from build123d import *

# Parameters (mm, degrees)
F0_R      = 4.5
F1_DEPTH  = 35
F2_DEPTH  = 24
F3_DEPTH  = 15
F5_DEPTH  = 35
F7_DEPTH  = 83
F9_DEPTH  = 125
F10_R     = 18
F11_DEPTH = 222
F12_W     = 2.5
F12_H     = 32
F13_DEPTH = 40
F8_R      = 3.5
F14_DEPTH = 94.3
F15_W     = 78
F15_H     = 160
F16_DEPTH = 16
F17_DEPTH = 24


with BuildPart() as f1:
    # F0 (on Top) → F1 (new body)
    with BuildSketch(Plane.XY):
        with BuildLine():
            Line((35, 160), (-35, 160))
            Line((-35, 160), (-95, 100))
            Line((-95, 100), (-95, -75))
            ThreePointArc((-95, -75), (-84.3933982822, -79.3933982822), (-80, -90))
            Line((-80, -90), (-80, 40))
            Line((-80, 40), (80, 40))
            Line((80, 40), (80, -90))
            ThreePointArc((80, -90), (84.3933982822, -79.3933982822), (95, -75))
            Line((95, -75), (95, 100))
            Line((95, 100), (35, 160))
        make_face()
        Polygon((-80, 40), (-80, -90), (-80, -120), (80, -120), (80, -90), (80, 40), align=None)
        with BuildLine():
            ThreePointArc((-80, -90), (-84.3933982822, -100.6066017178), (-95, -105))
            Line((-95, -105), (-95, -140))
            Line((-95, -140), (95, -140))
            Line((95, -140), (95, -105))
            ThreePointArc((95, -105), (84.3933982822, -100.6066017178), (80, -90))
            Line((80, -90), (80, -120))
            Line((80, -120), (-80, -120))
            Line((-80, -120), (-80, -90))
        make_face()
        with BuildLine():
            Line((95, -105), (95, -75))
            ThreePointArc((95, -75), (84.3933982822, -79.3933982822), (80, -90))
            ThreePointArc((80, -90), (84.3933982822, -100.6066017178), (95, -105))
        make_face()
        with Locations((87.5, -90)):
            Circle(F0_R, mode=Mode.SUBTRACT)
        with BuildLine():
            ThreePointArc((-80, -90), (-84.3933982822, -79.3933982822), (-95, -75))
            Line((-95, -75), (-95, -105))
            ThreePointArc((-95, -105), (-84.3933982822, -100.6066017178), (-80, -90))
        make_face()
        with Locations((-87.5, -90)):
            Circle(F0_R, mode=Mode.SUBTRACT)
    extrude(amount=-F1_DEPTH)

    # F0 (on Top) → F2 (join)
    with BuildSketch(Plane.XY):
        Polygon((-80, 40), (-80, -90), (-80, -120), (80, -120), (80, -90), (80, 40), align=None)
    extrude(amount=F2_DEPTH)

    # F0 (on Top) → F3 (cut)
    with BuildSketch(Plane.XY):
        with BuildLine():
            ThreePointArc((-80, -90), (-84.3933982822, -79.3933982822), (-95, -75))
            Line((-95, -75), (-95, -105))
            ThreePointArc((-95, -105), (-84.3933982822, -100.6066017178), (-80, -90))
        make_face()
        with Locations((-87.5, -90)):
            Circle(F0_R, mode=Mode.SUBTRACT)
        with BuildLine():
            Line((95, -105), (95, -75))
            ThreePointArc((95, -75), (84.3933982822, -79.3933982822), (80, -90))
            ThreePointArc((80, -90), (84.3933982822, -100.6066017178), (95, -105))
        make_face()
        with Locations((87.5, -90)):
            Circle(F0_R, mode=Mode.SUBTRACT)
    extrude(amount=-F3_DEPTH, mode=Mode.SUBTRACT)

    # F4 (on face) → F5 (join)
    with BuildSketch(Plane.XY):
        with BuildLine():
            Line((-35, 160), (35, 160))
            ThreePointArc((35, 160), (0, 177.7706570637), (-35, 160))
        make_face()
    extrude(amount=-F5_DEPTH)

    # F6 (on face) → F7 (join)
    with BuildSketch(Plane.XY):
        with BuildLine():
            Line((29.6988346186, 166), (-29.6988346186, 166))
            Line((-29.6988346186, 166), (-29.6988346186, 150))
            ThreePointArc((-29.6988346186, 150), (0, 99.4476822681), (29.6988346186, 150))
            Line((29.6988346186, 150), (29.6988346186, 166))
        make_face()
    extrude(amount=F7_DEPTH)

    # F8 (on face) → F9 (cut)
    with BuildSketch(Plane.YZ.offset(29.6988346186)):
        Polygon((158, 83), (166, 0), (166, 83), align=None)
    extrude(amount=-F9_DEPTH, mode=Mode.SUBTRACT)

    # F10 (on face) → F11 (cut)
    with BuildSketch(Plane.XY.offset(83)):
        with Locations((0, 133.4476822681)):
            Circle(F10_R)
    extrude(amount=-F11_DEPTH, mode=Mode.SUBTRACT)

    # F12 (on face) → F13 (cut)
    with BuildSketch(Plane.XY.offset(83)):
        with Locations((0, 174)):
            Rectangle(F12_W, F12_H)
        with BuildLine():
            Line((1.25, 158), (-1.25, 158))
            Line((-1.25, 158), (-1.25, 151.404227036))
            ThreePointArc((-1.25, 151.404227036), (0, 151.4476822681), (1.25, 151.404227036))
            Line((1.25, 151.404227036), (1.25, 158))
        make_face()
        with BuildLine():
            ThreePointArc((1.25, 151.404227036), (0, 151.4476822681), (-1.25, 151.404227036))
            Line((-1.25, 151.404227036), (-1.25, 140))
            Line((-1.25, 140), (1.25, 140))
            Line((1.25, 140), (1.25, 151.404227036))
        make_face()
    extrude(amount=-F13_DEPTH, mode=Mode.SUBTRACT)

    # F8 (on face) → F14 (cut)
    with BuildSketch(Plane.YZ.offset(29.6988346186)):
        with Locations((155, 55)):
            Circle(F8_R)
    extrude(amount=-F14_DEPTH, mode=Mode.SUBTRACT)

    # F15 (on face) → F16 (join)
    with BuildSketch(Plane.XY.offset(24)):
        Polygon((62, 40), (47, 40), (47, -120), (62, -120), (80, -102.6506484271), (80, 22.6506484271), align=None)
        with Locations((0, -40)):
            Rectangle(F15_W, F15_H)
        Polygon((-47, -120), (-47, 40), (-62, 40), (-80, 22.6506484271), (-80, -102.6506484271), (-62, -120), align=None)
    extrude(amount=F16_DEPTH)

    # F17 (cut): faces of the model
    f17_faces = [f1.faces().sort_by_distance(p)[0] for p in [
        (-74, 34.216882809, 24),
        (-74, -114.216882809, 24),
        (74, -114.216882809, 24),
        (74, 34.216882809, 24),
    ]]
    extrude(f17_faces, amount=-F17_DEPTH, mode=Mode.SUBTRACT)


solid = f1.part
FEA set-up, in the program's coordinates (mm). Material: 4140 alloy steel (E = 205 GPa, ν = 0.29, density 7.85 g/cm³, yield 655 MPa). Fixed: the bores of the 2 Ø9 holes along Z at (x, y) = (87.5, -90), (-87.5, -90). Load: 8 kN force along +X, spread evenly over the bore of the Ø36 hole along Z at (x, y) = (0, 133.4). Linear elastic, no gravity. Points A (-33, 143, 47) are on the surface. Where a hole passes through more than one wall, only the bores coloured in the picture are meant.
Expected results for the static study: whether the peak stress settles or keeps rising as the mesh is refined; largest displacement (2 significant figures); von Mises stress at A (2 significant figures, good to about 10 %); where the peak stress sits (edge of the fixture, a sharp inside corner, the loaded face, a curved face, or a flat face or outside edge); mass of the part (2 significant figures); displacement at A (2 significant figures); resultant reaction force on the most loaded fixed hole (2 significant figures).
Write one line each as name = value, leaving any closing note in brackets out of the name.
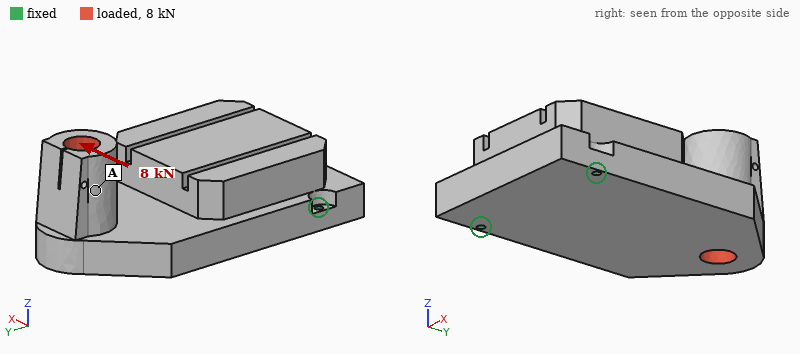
whether the peak stress settles or keeps rising as the mesh is refined = keeps rising
largest displacement = 38 µm
von Mises stress at A = 3.1 MPa
where the peak stress sits = edge of the fixture
mass of the part = 24 kg
displacement at A = 28 µm
resultant reaction force on the most loaded fixed hole = 11 kN
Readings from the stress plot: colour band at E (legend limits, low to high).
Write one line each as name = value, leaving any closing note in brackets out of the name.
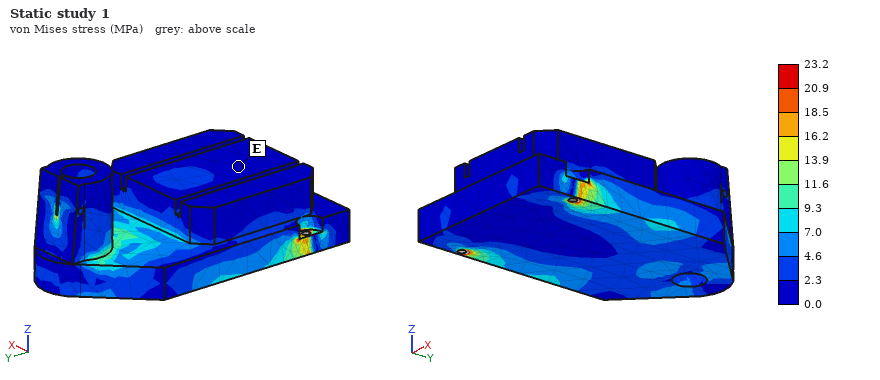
colour band at E = 0.0 to 2.3 MPa
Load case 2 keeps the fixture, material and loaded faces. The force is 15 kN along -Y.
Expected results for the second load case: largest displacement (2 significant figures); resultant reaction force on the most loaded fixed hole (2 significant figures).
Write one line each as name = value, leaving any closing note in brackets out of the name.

largest displacement = 0.27 mm
resultant reaction force on the most loaded fixed hole = 7.5 kN
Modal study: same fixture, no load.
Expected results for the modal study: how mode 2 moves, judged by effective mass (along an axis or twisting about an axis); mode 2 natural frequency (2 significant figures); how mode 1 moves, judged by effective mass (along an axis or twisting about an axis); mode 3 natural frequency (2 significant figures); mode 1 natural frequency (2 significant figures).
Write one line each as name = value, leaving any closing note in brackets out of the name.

how mode 2 moves, judged by effective mass = along X
mode 2 natural frequency = 1400 Hz
how mode 1 moves, judged by effective mass = along Z
mode 3 natural frequency = 1600 Hz
mode 1 natural frequency = 250 Hz
